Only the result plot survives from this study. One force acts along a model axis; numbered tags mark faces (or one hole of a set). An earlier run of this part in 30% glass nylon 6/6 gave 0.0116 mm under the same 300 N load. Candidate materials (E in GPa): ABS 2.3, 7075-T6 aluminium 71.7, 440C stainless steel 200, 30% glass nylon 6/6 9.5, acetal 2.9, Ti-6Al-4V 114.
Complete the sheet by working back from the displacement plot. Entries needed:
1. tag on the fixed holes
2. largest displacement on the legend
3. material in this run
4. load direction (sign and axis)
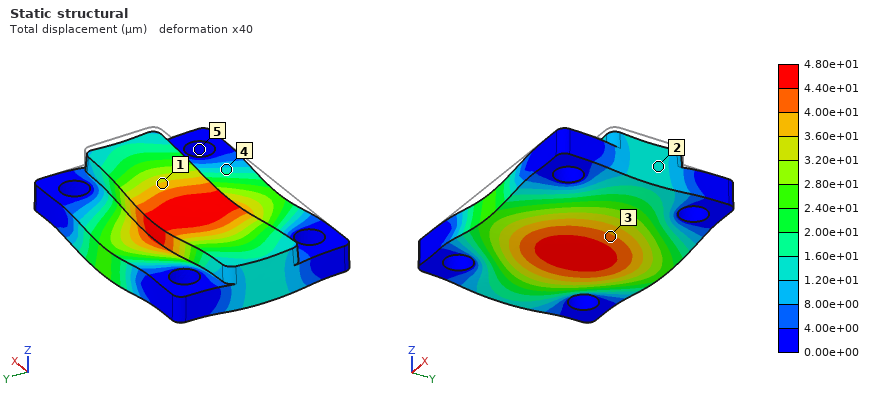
5
4.80e+01 µm
ABS
-Z
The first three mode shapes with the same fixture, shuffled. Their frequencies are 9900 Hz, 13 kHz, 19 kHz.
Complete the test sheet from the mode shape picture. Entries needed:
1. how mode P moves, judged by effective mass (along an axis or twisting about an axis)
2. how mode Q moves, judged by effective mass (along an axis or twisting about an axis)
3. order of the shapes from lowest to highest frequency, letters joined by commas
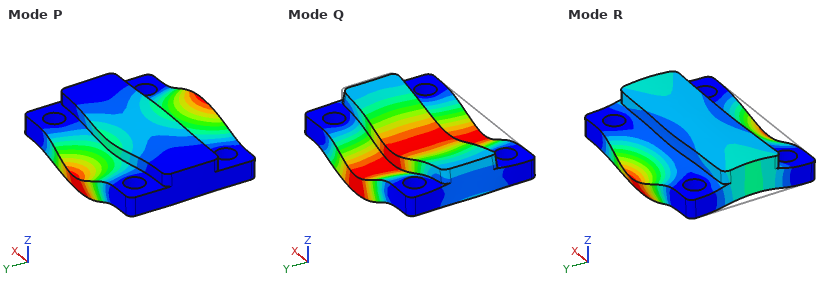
twisting about X
along Z
Q, P, R
